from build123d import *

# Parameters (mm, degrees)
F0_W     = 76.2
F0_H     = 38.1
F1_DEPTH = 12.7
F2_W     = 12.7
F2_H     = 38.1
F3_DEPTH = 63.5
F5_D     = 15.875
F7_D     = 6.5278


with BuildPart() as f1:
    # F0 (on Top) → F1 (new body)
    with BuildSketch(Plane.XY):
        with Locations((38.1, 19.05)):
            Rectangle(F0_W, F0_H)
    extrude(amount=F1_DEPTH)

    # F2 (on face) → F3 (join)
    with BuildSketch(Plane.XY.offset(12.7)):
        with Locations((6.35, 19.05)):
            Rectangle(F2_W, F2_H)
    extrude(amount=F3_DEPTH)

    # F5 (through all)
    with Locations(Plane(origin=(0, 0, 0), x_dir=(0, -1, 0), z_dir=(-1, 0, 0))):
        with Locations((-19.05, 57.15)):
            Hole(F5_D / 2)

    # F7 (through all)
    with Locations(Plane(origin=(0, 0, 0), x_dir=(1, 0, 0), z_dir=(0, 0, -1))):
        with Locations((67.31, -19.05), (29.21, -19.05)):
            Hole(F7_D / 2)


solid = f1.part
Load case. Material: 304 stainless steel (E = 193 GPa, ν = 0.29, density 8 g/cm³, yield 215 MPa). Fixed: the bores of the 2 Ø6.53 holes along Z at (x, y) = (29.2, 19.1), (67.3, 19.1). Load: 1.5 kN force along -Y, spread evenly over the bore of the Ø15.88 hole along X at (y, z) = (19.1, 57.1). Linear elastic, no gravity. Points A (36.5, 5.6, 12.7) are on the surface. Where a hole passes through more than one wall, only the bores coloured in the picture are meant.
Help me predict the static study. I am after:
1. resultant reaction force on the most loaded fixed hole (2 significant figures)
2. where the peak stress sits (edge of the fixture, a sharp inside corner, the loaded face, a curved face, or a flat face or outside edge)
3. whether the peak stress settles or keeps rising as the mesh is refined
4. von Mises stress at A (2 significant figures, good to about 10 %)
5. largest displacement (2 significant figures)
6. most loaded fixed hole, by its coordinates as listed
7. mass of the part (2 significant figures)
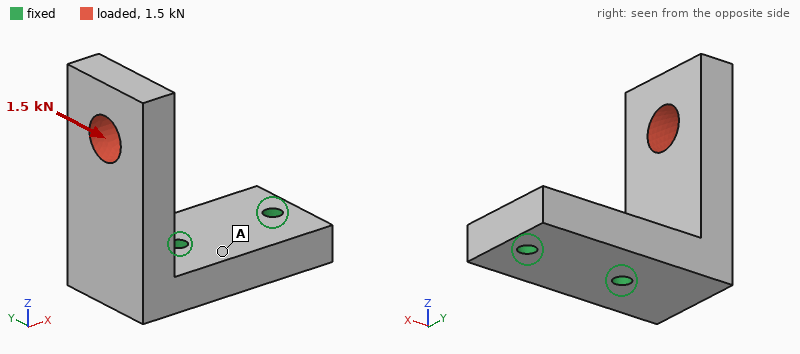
2.2 kN
edge of the fixture
keeps rising
18 MPa
84 µm
(29.2, 19.1)
510 g
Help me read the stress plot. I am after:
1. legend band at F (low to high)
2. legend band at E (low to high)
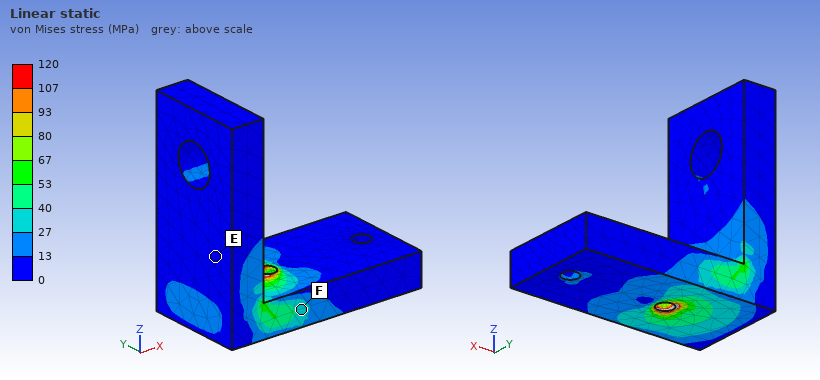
27 to 40 MPa
0 to 13 MPa
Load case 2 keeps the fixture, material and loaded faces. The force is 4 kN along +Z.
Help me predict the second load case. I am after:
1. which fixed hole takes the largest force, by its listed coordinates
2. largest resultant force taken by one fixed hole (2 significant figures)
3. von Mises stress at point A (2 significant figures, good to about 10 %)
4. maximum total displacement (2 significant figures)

(29.2, 19.1)
4.7 kN
26 MPa
75 µm
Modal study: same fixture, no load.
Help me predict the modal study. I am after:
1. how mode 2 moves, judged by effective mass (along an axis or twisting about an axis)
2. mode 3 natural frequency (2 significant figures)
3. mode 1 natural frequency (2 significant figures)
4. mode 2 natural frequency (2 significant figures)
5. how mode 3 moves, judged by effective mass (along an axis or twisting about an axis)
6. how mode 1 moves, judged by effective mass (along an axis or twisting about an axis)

along Y
5500 Hz
1400 Hz
2000 Hz
along Z
along X
